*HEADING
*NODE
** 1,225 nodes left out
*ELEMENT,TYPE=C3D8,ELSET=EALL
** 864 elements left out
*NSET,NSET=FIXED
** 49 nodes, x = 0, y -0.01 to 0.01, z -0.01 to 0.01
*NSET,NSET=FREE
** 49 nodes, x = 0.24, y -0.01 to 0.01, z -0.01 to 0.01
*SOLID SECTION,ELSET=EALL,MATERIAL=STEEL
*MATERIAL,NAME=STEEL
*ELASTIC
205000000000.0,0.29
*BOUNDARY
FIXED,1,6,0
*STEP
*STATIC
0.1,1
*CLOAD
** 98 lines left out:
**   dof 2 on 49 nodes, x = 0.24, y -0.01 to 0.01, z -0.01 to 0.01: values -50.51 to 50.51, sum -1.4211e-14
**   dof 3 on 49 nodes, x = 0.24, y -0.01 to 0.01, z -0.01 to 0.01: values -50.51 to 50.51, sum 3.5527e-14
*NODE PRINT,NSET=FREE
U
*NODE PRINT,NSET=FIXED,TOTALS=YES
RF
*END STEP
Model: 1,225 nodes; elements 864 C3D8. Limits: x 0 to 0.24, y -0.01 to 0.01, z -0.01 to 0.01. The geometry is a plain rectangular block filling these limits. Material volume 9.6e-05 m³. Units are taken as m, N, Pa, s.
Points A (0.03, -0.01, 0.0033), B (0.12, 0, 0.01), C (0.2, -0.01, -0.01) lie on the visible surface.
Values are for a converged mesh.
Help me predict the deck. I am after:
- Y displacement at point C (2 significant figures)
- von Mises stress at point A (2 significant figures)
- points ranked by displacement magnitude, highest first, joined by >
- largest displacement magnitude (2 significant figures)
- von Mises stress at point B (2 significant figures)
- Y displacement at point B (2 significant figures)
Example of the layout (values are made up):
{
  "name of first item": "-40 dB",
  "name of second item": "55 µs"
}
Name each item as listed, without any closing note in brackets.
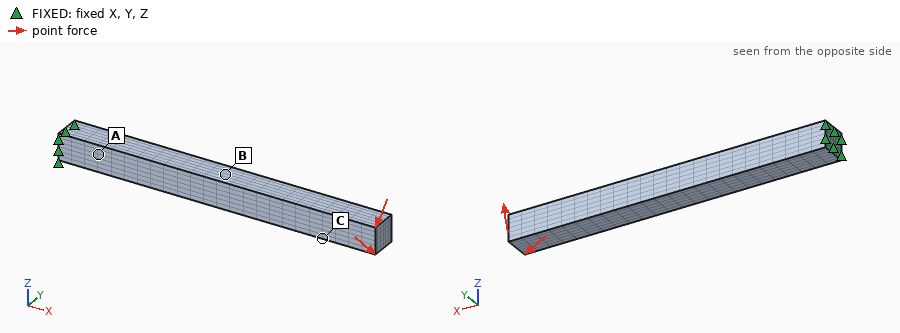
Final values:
{
  "Y displacement at point C": "2.5e-05 m",
  "von Mises stress at point A": "2.1e+07 Pa",
  "points ranked by displacement magnitude, highest first, joined by >": "C > B > A",
  "largest displacement magnitude": "4.5e-05 m",
  "von Mises stress at point B": "2.3e+07 Pa",
  "Y displacement at point B": "-1.5e-05 m"
}
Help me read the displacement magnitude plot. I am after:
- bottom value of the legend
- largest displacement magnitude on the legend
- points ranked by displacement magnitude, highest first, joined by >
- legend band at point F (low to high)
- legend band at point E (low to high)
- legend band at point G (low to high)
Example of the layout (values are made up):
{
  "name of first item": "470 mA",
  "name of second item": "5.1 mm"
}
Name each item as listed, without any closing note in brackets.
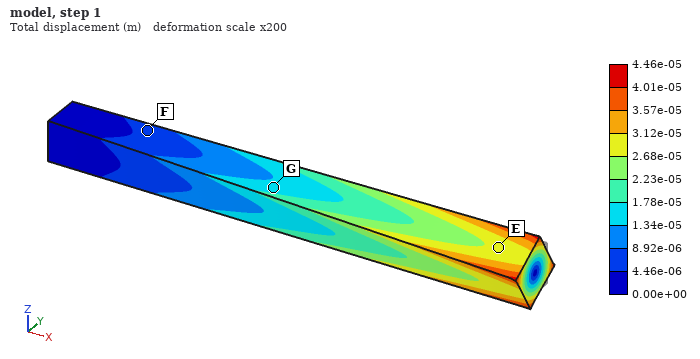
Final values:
{
  "bottom value of the legend": "0.00e+00 m",
  "largest displacement magnitude on the legend": "4.46e-05 m",
  "points ranked by displacement magnitude, highest first, joined by >": "E > G > F",
  "legend band at point F": "4.46e-06 to 8.92e-06 m",
  "legend band at point E": "2.68e-05 to 3.12e-05 m",
  "legend band at point G": "1.34e-05 to 1.78e-05 m"
}
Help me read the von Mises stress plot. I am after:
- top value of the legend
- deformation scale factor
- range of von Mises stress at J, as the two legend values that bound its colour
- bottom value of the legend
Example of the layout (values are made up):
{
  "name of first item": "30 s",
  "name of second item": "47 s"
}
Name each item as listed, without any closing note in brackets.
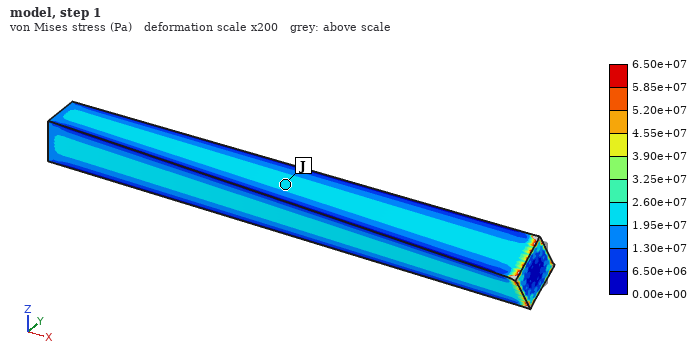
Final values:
{
  "top value of the legend": "6.50e+07 Pa",
  "deformation scale factor": "200",
  "range of von Mises stress at J, as the two legend values that bound its colour": "1.95e+07 to 2.60e+07 Pa",
  "bottom value of the legend": "0.00e+00 Pa"
}
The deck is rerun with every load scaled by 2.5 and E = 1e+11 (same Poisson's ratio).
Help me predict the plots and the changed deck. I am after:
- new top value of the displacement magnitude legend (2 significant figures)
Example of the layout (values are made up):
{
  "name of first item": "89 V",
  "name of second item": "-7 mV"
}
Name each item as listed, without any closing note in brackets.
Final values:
{
  "new top value of the displacement magnitude legend": "2.3e-04 m"
}
